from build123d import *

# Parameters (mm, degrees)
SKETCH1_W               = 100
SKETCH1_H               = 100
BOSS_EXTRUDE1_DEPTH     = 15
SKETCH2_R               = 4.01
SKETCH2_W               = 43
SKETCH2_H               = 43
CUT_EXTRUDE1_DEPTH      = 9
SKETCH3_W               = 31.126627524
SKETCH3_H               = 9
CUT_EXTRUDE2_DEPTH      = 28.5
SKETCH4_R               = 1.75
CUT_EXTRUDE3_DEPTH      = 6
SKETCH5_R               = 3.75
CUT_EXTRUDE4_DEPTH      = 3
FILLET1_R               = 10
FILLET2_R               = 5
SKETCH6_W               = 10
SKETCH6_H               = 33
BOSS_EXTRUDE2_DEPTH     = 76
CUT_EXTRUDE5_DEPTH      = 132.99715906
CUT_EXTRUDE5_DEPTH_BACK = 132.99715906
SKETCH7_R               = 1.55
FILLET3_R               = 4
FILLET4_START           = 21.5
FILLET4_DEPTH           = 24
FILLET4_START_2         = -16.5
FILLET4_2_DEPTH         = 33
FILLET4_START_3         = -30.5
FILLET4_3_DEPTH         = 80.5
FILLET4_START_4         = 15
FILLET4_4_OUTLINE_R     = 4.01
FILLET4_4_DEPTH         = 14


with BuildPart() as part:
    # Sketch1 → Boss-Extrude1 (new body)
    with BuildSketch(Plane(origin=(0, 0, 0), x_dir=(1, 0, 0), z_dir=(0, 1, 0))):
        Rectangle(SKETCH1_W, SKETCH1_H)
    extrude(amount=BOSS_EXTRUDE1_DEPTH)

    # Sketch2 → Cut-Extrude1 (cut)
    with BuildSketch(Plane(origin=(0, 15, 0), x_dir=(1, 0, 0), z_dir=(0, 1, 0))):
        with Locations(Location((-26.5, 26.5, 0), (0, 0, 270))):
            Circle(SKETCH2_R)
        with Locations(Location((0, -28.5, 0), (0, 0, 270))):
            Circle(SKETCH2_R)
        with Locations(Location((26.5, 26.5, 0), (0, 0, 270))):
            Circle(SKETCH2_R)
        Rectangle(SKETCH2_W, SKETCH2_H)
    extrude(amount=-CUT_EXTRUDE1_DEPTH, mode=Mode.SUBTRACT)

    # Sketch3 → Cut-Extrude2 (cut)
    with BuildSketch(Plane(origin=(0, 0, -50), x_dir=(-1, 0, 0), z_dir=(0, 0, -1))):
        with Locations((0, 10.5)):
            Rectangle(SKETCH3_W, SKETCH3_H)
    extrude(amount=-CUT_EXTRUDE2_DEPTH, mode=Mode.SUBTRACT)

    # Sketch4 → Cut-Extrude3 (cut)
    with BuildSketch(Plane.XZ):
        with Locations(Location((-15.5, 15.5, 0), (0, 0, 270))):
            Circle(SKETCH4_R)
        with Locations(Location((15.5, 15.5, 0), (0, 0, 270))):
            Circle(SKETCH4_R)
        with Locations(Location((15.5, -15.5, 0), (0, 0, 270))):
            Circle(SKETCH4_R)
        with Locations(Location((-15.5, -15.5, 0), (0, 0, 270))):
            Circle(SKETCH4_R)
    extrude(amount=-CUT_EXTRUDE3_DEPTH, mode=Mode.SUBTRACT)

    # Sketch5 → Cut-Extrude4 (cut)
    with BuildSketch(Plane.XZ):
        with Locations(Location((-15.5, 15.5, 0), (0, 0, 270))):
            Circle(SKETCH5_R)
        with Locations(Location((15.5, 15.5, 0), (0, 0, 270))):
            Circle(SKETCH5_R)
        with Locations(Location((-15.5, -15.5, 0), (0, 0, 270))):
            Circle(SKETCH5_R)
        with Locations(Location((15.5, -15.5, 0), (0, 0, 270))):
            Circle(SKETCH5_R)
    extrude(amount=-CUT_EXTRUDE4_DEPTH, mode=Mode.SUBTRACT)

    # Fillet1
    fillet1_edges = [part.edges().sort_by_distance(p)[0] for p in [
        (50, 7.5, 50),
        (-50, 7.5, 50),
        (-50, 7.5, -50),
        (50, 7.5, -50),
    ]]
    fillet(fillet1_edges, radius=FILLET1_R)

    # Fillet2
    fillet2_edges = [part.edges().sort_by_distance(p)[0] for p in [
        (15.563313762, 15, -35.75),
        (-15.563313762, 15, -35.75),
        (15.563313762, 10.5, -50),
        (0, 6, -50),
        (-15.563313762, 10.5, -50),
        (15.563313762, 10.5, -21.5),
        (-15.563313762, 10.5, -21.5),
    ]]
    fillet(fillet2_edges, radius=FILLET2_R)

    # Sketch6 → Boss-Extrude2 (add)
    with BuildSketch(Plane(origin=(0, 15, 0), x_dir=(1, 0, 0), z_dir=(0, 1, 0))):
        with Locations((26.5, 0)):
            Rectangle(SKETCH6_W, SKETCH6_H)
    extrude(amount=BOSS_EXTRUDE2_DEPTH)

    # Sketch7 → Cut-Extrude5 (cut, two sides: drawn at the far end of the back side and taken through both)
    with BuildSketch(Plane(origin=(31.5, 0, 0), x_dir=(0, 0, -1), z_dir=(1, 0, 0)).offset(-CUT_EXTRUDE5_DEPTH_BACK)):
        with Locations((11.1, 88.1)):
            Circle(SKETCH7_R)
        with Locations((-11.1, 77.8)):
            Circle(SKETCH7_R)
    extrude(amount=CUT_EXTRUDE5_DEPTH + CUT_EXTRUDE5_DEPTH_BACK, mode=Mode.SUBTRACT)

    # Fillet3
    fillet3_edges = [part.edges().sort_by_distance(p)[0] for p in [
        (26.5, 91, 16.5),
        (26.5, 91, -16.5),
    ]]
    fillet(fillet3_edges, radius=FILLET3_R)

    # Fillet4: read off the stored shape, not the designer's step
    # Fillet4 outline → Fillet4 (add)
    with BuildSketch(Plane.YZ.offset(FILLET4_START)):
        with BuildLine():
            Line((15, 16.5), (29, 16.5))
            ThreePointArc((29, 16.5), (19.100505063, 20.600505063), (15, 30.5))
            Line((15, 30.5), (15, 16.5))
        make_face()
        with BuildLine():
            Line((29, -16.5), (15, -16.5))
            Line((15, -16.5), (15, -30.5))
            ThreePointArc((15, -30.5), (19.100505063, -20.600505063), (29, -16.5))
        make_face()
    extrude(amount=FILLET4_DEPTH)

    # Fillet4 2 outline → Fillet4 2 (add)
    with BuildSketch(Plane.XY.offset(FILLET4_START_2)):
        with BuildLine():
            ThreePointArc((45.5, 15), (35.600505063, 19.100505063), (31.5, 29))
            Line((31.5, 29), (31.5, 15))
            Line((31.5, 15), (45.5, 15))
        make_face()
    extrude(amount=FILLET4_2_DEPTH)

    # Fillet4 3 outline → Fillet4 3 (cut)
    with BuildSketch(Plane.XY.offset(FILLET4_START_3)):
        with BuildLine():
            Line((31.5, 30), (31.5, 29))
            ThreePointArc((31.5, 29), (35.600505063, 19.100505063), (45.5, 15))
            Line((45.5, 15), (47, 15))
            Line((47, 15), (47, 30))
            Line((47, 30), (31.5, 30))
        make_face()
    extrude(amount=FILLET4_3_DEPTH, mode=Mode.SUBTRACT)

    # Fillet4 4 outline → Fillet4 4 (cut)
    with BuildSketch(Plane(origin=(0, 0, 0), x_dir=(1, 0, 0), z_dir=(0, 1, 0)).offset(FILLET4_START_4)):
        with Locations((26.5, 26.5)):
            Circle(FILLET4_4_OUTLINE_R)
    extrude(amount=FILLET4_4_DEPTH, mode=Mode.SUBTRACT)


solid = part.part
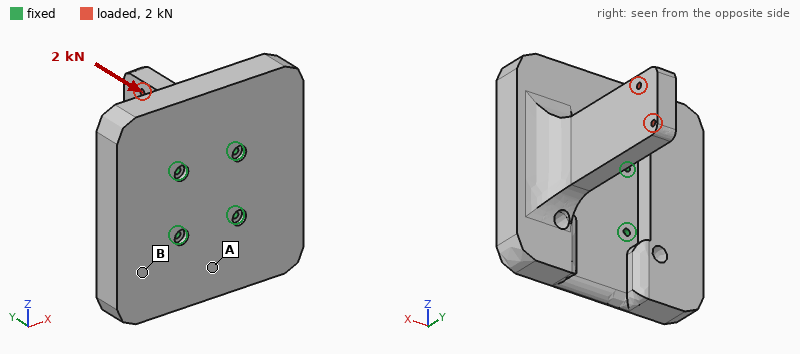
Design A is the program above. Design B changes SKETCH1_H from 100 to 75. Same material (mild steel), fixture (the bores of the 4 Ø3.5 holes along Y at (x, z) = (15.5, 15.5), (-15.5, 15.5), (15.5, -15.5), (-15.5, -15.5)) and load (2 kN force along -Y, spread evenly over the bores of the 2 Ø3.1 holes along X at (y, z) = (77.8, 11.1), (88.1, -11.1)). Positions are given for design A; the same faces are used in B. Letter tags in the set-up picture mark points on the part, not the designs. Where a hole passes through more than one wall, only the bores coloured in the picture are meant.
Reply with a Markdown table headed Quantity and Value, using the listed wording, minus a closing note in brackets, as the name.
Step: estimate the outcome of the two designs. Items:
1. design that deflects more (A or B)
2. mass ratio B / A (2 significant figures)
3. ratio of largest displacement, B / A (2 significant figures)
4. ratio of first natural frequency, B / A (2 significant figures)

| Quantity | Value |
|---|---|
| design that deflects more | B |
| mass ratio B / A | 0.77 |
| ratio of largest displacement, B / A | 1.2 |
| ratio of first natural frequency, B / A | 0.94 |
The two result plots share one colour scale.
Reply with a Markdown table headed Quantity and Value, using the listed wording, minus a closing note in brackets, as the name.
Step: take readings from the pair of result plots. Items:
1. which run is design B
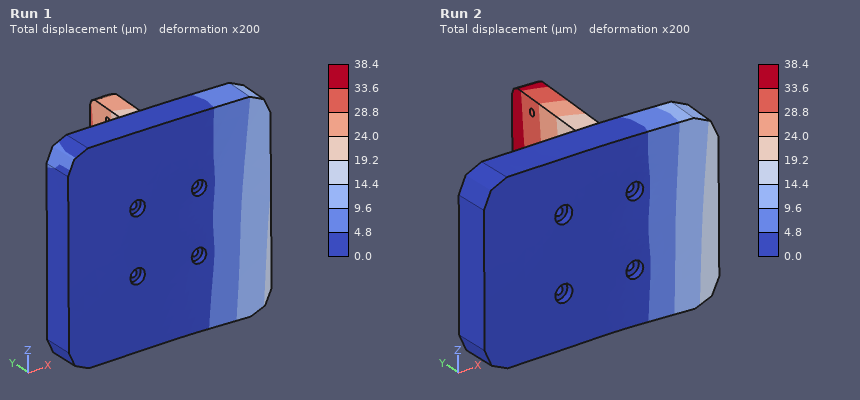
| Quantity | Value |
|---|---|
| which run is design B | Run 2 |
